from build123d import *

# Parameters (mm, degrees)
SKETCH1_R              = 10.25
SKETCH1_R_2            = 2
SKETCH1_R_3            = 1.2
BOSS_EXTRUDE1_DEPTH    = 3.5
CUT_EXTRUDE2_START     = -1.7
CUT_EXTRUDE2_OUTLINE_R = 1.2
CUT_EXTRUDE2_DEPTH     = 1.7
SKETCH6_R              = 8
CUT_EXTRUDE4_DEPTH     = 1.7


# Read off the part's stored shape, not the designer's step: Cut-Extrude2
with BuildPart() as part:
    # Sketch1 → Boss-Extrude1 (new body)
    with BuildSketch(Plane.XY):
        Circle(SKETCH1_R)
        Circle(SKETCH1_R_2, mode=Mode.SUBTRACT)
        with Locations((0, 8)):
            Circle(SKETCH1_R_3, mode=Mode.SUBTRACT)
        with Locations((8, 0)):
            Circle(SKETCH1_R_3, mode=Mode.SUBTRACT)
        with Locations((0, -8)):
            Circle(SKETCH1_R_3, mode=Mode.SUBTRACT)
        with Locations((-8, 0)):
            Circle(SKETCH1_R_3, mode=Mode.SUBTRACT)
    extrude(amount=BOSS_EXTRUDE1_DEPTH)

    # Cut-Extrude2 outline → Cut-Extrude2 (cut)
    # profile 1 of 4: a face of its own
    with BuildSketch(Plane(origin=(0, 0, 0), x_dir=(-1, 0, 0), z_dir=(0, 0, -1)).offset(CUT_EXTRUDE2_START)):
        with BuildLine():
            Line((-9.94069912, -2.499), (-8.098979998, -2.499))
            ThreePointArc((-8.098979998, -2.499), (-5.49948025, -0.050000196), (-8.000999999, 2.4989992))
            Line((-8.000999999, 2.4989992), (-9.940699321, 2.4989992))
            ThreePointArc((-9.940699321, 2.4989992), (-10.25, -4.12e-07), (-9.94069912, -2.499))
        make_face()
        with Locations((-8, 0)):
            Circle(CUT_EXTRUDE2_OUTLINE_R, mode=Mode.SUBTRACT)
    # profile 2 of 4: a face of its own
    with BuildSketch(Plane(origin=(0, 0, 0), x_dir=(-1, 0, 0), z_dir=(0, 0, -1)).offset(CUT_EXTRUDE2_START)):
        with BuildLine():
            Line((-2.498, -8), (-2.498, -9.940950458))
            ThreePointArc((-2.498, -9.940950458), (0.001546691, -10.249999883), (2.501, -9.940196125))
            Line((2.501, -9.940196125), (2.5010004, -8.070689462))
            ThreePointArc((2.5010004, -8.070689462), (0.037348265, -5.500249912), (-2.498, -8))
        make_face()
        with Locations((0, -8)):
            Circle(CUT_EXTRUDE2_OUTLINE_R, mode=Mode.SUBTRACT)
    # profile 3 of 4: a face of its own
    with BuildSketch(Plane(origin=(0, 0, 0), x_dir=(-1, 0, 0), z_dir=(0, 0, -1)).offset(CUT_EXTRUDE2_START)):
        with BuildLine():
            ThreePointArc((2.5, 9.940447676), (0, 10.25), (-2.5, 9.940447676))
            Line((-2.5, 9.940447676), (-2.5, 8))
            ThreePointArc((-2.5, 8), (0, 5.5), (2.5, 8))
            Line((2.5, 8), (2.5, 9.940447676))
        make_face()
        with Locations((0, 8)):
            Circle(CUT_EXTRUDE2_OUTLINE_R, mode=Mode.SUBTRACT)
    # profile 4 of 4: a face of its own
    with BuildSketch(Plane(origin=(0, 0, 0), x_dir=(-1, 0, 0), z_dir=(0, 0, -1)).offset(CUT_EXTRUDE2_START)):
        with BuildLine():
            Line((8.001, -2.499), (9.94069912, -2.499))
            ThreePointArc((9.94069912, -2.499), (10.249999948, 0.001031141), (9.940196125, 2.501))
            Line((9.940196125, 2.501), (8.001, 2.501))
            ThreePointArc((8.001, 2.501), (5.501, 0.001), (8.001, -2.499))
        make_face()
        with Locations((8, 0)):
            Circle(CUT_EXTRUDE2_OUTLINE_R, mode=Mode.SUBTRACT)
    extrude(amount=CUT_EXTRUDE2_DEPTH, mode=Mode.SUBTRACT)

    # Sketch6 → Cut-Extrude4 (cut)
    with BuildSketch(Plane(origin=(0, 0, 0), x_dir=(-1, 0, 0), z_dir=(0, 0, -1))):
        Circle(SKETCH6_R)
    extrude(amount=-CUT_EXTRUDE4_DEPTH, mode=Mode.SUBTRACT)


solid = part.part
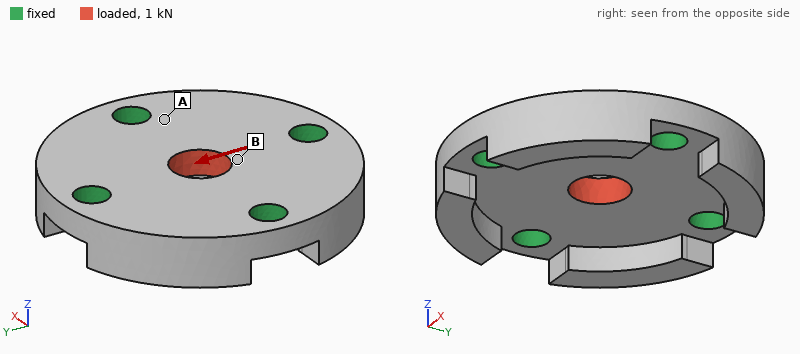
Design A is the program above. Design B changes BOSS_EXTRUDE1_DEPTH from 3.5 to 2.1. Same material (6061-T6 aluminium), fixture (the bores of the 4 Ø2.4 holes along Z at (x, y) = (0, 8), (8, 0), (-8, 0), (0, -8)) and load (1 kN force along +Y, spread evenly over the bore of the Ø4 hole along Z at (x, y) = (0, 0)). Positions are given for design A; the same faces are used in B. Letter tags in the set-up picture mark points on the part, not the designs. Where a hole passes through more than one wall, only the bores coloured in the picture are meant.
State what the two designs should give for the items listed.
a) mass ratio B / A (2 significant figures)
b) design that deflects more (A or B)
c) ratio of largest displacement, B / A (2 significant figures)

0.38
B
4.4
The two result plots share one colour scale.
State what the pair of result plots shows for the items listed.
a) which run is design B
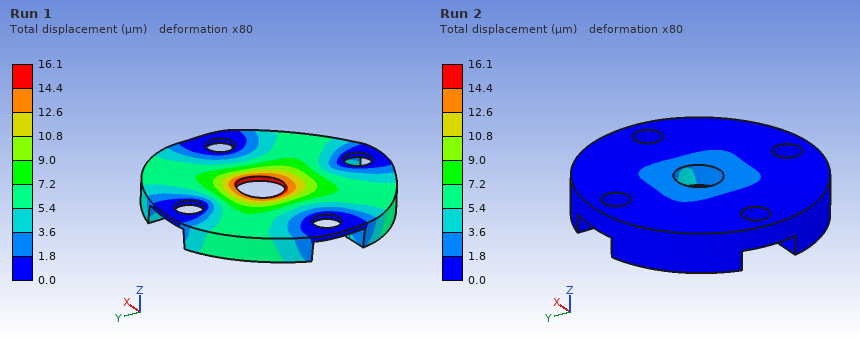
Run 1
